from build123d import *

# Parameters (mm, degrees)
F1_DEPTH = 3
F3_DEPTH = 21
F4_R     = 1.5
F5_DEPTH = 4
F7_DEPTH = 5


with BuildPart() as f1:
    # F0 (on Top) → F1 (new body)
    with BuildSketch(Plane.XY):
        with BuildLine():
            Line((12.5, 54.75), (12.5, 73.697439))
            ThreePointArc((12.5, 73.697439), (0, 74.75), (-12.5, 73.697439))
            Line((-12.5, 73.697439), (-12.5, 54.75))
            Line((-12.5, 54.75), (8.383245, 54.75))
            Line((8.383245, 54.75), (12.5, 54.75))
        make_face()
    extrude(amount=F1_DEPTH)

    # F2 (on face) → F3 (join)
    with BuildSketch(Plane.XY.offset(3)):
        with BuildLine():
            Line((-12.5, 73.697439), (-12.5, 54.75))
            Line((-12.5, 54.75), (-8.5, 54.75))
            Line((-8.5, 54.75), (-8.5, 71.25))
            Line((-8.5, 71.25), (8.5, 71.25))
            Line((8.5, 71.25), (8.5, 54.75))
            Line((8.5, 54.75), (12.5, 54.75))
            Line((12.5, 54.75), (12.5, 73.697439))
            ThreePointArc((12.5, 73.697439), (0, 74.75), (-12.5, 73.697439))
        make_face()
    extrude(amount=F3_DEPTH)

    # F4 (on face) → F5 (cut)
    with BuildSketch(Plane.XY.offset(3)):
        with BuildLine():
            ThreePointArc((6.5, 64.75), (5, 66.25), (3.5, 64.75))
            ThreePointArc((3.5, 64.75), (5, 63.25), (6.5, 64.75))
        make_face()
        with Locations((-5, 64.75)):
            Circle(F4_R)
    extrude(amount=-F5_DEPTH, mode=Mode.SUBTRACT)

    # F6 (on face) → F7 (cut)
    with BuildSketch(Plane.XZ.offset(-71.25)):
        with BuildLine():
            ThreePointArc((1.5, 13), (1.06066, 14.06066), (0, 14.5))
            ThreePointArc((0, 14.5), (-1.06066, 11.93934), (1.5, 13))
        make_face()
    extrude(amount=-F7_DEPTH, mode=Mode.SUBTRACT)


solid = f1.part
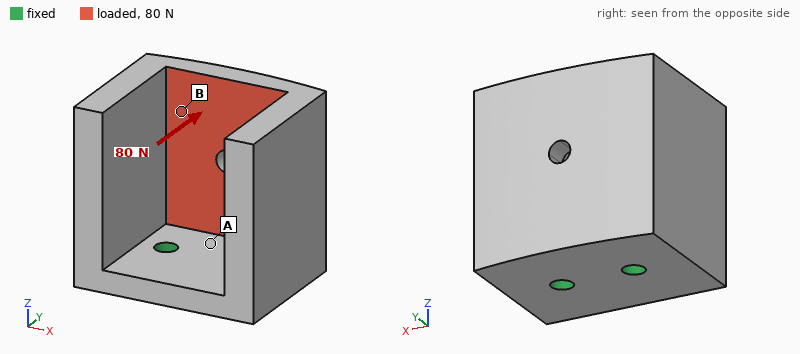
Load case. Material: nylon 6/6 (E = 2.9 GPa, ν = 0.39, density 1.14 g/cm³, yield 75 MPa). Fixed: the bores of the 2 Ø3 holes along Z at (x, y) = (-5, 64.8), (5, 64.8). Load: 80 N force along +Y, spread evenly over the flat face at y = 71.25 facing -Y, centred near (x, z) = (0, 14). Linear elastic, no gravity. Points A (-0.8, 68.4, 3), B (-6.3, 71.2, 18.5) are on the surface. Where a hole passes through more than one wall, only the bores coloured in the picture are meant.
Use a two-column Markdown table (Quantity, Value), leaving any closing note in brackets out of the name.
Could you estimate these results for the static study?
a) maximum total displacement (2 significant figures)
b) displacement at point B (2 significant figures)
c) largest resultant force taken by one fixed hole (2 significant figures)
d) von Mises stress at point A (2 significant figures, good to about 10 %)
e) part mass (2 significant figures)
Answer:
| Quantity | Value |
|---|---|
| maximum total displacement | 0.30 mm |
| displacement at point B | 0.21 mm |
| largest resultant force taken by one fixed hole | 41 N |
| von Mises stress at point A | 6.8 MPa |
| part mass | 6.6 g |
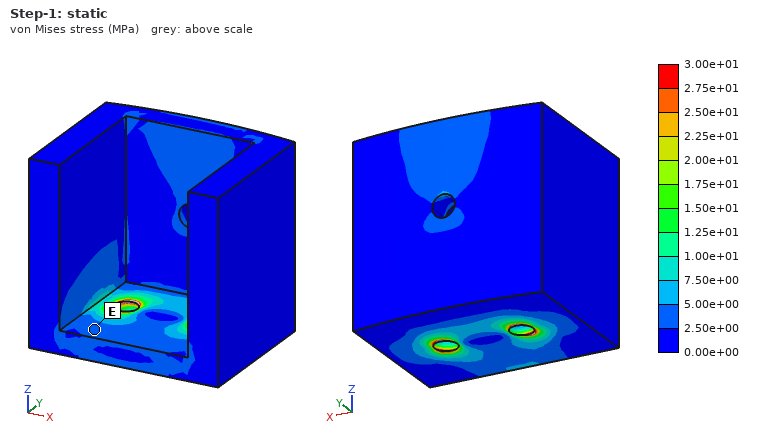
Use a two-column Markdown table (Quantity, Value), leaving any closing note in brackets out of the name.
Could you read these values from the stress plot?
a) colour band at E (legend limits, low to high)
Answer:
| Quantity | Value |
|---|---|
| colour band at E | 2.50e+00 to 5.00e+00 MPa |
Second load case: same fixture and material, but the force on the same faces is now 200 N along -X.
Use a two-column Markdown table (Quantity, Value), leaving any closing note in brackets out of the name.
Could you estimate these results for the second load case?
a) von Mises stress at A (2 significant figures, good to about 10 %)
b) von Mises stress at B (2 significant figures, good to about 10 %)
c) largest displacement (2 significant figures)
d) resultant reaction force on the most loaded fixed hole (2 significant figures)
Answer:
| Quantity | Value |
|---|---|
| von Mises stress at A | 15 MPa |
| von Mises stress at B | 8.7 MPa |
| largest displacement | 0.44 mm |
| resultant reaction force on the most loaded fixed hole | 210 N |
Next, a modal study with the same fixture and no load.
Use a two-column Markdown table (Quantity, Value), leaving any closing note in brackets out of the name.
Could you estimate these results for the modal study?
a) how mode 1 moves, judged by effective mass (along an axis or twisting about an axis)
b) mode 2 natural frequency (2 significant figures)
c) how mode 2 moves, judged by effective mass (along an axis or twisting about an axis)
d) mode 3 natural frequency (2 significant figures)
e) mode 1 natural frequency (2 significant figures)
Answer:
| Quantity | Value |
|---|---|
| how mode 1 moves, judged by effective mass | along Y |
| mode 2 natural frequency | 1600 Hz |
| how mode 2 moves, judged by effective mass | along X |
| mode 3 natural frequency | 3100 Hz |
| mode 1 natural frequency | 1400 Hz |
